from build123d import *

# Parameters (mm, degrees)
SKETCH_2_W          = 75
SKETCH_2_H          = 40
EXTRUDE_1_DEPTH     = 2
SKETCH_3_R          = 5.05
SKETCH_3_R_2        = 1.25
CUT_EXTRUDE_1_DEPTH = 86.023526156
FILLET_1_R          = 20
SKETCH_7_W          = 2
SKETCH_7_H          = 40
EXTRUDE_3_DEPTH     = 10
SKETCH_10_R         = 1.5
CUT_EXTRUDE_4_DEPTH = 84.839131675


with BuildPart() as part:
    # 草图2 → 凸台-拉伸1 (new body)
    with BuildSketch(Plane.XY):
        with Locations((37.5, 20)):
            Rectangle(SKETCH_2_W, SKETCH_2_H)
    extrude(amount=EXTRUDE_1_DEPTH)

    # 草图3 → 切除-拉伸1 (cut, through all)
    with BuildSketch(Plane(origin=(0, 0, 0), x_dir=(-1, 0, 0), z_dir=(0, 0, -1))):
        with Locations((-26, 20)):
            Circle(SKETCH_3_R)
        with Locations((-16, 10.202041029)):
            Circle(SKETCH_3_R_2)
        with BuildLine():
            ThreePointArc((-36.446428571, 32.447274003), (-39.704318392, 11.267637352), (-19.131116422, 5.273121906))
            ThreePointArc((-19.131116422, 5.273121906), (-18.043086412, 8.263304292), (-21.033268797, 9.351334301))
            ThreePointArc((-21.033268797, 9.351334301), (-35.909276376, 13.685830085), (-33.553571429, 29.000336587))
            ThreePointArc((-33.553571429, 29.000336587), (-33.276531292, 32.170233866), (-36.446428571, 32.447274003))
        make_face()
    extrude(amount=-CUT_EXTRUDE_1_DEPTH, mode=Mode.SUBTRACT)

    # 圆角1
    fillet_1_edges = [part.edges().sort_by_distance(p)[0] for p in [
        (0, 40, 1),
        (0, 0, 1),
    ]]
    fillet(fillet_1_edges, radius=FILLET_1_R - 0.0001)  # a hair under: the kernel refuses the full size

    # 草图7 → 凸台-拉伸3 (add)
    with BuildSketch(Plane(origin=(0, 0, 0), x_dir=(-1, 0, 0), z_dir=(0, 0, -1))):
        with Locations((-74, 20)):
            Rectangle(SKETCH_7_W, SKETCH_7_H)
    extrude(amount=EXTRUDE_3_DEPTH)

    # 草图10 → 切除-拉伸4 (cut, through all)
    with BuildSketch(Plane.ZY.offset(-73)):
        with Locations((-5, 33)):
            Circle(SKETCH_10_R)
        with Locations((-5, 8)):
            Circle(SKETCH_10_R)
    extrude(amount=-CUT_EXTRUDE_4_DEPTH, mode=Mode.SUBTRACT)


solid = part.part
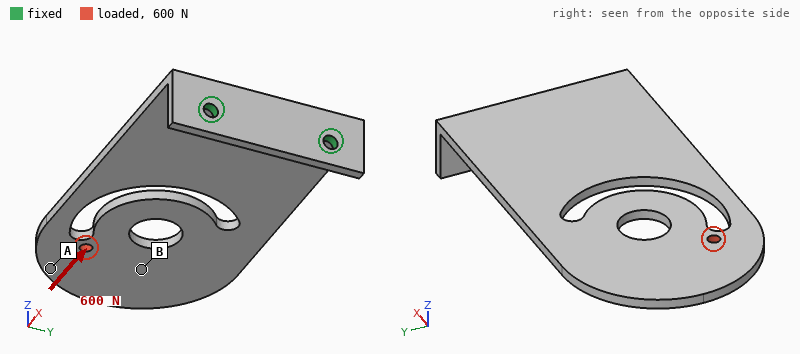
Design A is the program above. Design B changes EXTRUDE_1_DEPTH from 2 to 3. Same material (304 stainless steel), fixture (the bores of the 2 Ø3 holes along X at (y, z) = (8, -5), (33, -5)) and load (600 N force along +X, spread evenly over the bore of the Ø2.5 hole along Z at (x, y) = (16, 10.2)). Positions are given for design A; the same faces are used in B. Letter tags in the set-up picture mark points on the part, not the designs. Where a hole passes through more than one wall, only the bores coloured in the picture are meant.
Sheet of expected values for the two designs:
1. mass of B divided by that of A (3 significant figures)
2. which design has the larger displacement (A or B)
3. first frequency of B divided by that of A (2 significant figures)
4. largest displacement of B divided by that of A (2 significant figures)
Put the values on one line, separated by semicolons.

1.43; B; 1.2; 1.1
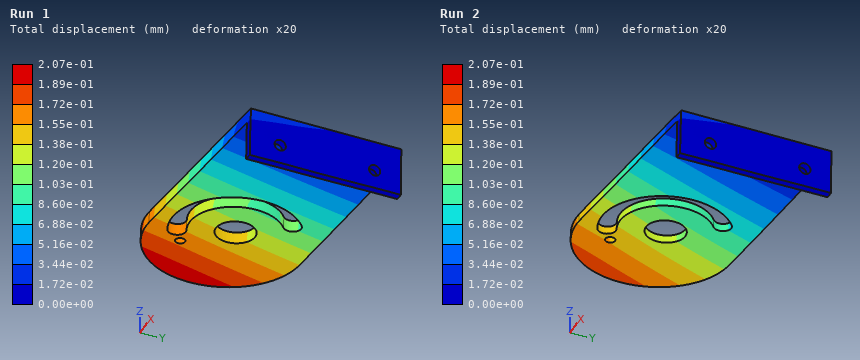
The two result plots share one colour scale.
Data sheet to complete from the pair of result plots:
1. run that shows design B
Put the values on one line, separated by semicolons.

Run 1
